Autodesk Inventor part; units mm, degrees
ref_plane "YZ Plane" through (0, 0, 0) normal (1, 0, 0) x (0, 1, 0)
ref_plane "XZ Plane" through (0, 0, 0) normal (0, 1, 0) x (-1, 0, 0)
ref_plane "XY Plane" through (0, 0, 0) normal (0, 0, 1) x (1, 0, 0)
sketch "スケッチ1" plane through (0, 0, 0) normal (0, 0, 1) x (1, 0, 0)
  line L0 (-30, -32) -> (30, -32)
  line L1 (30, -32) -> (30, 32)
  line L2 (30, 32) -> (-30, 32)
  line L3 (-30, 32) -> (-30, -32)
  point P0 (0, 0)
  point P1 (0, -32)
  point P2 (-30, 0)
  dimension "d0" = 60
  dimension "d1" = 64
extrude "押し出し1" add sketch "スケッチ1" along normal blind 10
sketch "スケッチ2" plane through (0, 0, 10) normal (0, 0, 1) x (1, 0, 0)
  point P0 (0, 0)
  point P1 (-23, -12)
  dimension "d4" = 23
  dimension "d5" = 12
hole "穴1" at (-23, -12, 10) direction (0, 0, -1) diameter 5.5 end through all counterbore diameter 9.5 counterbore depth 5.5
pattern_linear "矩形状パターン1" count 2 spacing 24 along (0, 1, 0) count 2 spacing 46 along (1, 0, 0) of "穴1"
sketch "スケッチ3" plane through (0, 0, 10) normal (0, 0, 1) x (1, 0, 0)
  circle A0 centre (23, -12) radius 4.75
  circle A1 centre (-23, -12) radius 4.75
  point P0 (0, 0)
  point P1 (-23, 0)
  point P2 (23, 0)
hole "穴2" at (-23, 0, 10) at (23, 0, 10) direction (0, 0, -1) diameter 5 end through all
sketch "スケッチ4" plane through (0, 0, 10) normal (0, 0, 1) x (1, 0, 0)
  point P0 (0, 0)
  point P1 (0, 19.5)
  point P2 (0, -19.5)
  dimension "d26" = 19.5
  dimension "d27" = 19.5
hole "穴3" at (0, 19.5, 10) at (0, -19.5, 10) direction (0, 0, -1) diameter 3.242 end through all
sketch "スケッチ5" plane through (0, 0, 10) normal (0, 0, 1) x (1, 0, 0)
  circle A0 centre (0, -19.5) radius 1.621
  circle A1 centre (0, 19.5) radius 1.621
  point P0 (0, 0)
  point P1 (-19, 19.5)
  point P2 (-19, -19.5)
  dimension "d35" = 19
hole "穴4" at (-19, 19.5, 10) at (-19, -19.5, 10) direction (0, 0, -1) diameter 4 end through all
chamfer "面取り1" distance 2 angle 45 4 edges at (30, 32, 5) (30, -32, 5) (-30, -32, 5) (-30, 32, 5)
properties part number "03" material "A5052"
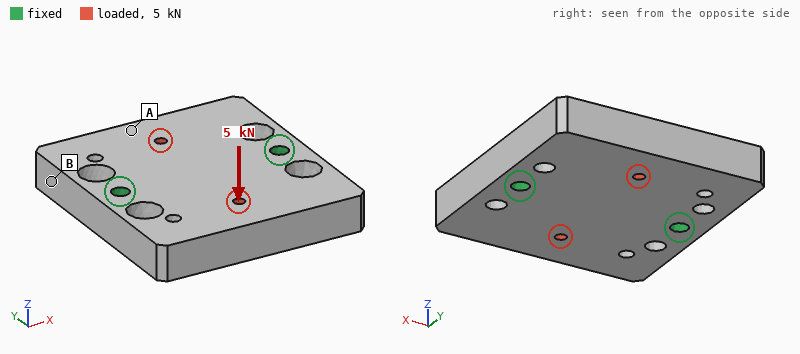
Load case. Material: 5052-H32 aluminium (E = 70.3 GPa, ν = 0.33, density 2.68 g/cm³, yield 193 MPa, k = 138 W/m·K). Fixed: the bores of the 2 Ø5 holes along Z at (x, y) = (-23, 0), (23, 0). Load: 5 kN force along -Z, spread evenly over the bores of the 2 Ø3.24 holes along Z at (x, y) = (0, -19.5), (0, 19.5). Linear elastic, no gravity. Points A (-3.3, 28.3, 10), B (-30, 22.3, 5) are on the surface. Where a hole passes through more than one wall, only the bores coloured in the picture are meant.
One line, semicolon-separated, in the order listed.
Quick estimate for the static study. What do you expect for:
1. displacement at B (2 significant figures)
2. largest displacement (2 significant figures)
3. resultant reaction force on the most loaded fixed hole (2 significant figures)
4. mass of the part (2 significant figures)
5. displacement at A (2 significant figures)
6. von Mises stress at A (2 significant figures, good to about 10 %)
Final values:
19 µm; 61 µm; 2.5 kN; 95 g; 54 µm; 32 MPa
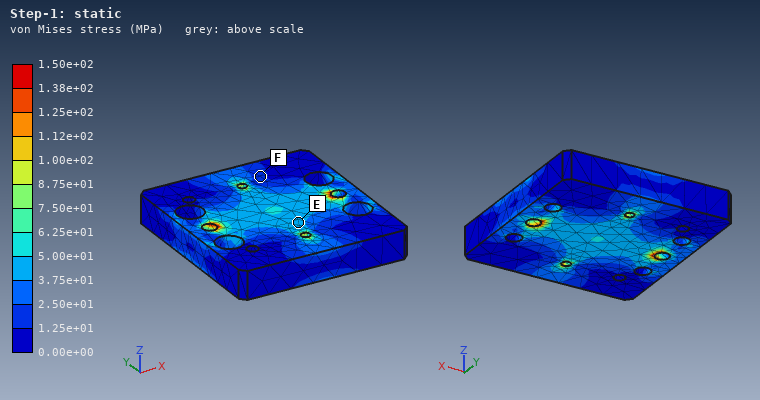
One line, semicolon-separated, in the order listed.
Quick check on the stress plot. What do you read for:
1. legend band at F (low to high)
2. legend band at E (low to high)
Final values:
1.25e+01 to 2.50e+01 MPa; 3.75e+01 to 5.00e+01 MPa
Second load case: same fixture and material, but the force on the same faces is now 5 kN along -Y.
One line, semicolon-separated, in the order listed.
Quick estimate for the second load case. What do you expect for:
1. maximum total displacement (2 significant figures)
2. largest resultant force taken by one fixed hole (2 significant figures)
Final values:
7.7 µm; 2.5 kN
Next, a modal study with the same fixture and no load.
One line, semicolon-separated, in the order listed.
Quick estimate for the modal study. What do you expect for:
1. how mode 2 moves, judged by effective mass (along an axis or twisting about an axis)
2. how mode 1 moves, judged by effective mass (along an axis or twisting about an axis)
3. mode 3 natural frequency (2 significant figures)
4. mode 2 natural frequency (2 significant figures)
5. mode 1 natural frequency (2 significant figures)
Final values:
along Z; twisting about X; 10 kHz; 6900 Hz; 4900 Hz
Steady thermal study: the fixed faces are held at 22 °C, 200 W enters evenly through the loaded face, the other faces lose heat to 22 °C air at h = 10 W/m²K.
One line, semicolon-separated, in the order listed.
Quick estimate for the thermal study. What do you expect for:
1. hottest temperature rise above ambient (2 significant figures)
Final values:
69 K
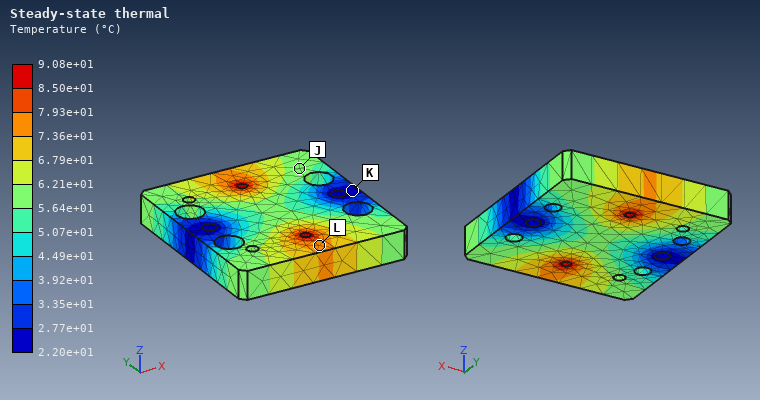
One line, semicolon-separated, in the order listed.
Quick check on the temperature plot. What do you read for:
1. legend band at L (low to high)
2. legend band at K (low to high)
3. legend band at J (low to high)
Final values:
7.36e+01 to 7.93e+01 °C; 2.20e+01 to 2.77e+01 °C; 5.64e+01 to 6.21e+01 °C
